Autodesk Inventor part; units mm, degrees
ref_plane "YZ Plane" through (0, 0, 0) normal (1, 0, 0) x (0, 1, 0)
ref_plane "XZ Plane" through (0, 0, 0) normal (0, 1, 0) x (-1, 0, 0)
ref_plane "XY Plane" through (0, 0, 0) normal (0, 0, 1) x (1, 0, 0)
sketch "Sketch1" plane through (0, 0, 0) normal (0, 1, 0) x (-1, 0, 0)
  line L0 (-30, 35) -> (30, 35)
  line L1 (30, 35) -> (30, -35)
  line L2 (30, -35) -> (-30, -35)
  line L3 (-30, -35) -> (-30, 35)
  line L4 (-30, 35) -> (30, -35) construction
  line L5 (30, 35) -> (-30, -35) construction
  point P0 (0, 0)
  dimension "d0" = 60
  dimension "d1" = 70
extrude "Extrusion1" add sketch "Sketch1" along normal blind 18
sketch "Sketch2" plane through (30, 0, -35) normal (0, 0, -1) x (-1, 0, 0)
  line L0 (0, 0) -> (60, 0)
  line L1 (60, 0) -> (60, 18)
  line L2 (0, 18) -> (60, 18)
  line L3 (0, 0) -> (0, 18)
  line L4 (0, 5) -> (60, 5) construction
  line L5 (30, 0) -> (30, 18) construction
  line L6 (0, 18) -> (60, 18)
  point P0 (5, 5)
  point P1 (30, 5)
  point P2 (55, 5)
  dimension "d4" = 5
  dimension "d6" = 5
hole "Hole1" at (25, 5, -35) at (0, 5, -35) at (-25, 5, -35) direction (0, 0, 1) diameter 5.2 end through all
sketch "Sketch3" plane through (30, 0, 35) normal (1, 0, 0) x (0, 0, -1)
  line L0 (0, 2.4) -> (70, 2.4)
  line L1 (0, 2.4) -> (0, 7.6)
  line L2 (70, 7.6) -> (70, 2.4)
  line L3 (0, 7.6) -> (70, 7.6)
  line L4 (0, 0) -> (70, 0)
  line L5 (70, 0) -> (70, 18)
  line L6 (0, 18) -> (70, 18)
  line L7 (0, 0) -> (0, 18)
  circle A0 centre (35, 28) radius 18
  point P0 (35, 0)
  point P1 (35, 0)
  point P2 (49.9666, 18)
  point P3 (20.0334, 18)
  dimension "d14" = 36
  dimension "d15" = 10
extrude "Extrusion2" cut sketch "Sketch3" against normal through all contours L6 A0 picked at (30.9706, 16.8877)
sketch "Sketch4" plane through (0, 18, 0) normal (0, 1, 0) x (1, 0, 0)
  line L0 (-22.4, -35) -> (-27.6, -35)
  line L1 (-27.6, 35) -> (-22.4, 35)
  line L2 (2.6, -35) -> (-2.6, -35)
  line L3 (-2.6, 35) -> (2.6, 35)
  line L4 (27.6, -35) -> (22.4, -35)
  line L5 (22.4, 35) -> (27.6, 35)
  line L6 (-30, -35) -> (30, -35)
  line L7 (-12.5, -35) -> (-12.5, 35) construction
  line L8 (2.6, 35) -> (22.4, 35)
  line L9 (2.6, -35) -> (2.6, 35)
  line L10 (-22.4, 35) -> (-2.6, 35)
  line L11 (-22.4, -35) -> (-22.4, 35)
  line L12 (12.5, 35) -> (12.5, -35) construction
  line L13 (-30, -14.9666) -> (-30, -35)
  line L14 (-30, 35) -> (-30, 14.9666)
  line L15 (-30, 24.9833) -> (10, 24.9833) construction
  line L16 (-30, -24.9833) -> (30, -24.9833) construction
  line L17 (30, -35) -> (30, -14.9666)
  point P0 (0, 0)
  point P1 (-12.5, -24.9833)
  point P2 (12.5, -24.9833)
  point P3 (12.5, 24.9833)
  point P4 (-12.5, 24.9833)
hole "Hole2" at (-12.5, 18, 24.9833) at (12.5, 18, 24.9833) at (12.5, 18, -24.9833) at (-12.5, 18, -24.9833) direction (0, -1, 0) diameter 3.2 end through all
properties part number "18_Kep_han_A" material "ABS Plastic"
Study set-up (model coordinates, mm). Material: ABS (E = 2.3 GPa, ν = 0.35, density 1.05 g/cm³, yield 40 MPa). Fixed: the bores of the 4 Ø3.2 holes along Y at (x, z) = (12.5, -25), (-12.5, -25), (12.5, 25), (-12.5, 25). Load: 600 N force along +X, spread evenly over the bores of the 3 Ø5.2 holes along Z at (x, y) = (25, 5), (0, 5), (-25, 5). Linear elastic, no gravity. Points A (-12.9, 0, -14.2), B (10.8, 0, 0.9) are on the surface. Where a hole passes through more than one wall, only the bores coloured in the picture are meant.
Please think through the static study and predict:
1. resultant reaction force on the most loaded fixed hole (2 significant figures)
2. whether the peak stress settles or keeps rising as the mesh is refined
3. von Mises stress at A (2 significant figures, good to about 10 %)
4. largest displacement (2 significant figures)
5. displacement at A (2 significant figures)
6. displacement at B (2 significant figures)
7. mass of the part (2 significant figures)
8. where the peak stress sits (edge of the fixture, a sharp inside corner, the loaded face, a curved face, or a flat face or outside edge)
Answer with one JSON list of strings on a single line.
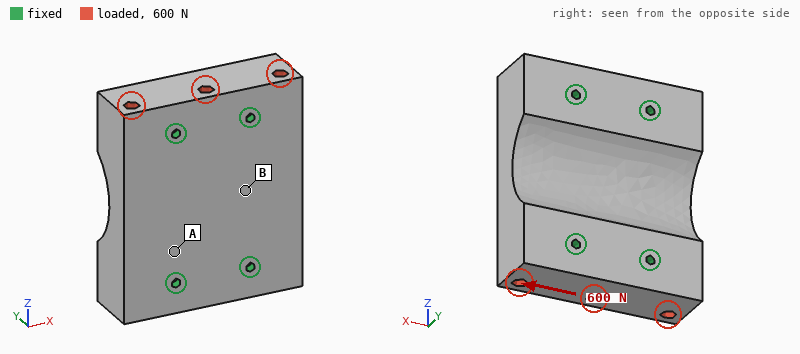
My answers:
["150 N", "keeps rising", "0.37 MPa", "10 µm", "5.4 µm", "7.6 µm", "63 g", "edge of the fixture"]
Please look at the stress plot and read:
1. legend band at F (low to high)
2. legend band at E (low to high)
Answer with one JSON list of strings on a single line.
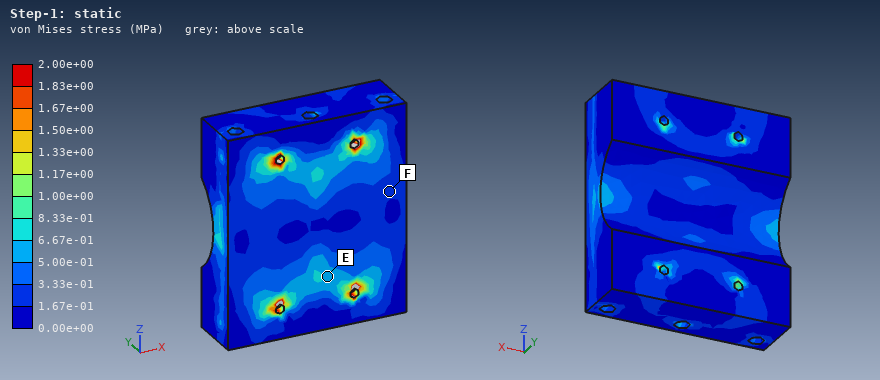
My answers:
["1.67e-01 to 3.33e-01 MPa", "5.00e-01 to 6.67e-01 MPa"]
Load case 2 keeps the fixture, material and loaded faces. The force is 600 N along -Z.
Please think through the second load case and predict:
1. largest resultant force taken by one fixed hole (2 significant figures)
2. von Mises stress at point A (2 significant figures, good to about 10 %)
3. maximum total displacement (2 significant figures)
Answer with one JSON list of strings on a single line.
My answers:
["150 N", "0.31 MPa", "8.5 µm"]
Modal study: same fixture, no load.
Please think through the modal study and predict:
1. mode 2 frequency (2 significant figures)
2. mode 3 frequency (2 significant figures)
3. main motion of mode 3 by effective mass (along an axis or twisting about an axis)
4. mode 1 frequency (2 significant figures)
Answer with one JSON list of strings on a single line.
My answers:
["5400 Hz", "7500 Hz", "along X", "5400 Hz"]
